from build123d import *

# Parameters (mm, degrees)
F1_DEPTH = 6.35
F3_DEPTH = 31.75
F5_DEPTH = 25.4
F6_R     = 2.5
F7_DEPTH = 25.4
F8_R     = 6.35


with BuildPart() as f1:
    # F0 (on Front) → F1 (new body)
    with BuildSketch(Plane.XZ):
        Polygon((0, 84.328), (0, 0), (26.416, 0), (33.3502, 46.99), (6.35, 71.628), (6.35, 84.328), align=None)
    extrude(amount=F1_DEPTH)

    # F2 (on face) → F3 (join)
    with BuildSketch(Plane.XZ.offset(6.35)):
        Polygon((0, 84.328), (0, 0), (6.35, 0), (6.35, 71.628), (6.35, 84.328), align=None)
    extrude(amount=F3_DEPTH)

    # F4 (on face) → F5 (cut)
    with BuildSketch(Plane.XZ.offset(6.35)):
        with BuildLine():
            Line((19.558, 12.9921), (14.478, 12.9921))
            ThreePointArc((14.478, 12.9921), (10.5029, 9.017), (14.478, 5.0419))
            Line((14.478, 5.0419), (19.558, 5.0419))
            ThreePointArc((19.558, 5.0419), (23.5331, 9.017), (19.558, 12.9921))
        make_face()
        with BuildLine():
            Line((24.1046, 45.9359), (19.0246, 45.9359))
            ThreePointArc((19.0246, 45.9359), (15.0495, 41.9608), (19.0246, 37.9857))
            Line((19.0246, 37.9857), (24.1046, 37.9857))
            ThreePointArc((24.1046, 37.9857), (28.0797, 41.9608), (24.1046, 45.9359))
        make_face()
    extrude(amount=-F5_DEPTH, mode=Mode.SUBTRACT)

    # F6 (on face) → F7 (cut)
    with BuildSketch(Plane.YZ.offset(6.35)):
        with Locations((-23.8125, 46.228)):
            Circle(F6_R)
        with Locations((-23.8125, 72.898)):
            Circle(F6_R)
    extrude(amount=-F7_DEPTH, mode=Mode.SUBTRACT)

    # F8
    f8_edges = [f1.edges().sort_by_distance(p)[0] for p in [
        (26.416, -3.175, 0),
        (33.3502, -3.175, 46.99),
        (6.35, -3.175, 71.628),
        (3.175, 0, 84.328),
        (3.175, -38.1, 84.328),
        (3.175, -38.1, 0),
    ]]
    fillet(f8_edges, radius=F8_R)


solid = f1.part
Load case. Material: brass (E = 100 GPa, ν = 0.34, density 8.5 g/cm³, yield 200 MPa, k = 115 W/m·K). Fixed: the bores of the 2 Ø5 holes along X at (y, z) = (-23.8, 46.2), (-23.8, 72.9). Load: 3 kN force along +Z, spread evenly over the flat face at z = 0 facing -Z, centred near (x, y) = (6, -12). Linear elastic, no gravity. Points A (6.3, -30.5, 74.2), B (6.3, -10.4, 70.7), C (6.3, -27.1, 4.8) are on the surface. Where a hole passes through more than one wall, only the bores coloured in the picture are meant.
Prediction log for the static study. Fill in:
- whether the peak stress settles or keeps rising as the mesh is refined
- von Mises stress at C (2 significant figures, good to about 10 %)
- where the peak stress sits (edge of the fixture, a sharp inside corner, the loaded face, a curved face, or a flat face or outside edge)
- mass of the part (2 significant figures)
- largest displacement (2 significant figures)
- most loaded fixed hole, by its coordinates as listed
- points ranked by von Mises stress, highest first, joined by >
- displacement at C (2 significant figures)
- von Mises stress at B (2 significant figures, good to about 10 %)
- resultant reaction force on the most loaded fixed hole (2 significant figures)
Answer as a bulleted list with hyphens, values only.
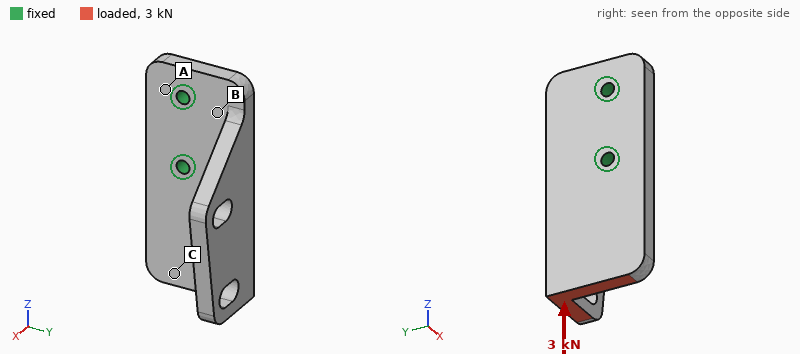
- keeps rising
- 9.4 MPa
- edge of the fixture
- 240 g
- 38 µm
- (-23.8, 46.2)
- B > C > A
- 18 µm
- 19 MPa
- 2.3 kN
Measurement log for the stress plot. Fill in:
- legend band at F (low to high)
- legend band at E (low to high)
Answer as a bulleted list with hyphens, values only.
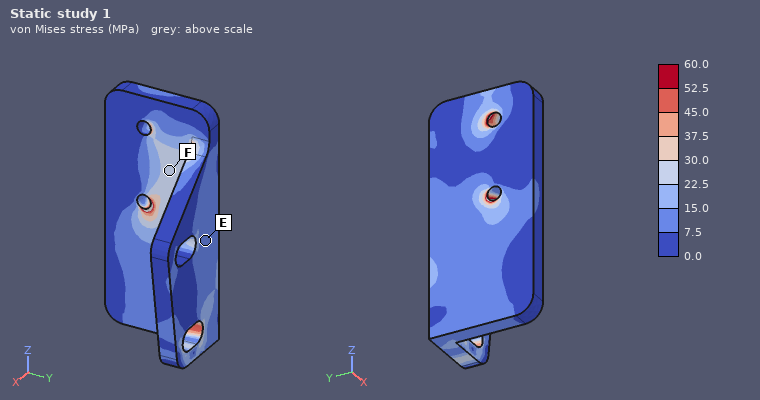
- 22.5 to 30.0 MPa
- 7.5 to 15.0 MPa
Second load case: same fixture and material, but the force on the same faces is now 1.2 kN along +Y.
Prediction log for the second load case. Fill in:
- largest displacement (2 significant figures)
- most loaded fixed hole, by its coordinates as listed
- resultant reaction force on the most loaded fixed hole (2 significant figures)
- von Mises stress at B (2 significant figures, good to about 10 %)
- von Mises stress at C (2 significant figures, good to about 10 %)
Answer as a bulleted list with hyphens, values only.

- 83 µm
- (-23.8, 46.2)
- 2.9 kN
- 11 MPa
- 12 MPa
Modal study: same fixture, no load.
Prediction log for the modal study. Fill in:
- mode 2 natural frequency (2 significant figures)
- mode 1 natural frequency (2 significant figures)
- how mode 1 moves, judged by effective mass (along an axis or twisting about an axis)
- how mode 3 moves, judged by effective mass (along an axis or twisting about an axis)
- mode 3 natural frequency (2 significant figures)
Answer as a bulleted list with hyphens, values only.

- 2300 Hz
- 1500 Hz
- along X
- along Y
- 3900 Hz
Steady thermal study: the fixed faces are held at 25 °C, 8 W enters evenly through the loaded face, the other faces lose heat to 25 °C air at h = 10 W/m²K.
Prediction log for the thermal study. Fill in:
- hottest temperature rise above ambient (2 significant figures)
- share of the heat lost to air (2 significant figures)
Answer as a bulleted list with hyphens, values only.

- 13 K
- 6.0 %
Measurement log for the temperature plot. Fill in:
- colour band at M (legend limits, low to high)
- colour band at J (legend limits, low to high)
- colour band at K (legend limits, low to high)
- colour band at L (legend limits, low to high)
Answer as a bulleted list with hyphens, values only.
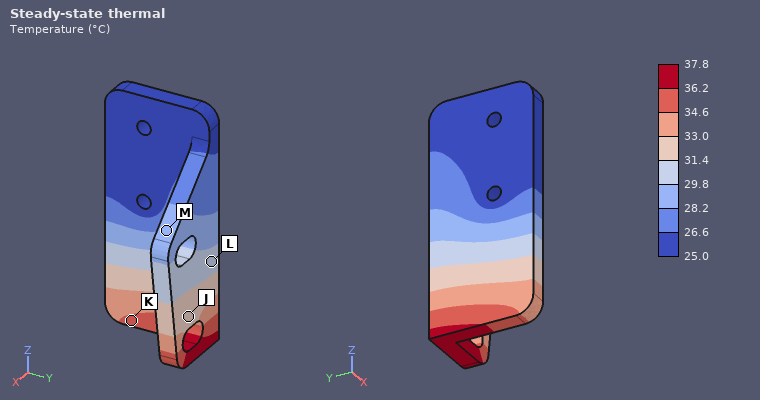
- 28.2 to 29.8 °C
- 31.4 to 33.0 °C
- 34.6 to 36.2 °C
- 29.8 to 31.4 °C
